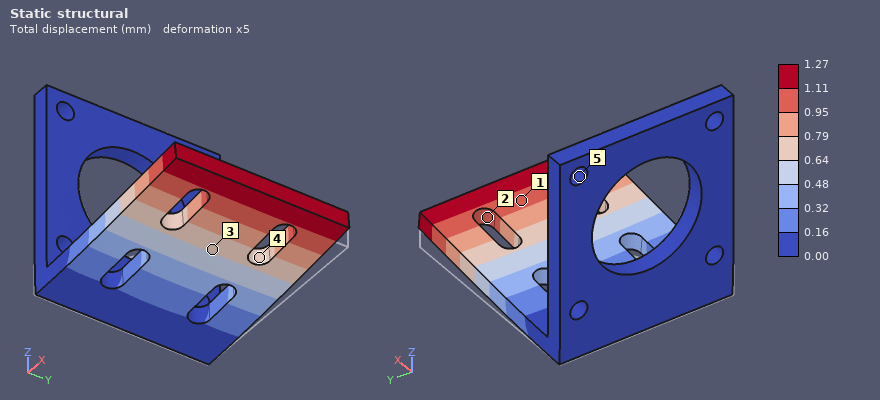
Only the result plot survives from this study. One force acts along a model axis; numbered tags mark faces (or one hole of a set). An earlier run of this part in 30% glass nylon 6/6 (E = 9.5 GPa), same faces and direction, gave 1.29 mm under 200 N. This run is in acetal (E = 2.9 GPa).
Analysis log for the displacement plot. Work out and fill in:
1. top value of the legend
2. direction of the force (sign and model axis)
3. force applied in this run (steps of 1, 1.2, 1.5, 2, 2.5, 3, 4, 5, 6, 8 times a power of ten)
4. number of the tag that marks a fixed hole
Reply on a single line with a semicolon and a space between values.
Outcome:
1.27 mm; +Z; 60 N; 5
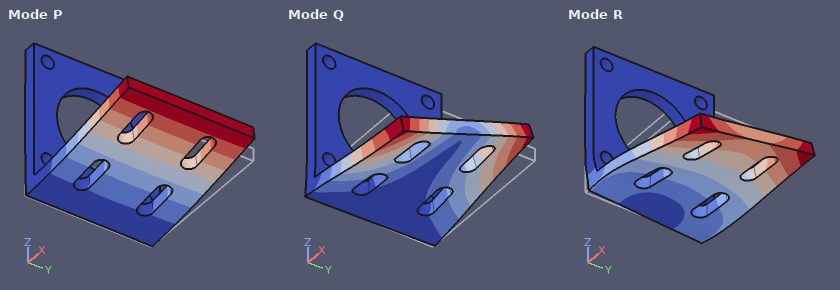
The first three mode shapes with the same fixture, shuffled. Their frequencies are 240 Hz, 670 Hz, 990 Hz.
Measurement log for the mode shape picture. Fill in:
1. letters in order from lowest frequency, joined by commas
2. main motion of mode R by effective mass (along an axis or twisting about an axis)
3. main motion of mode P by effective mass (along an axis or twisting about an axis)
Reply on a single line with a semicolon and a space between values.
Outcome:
P, Q, R; along Y; along Z
